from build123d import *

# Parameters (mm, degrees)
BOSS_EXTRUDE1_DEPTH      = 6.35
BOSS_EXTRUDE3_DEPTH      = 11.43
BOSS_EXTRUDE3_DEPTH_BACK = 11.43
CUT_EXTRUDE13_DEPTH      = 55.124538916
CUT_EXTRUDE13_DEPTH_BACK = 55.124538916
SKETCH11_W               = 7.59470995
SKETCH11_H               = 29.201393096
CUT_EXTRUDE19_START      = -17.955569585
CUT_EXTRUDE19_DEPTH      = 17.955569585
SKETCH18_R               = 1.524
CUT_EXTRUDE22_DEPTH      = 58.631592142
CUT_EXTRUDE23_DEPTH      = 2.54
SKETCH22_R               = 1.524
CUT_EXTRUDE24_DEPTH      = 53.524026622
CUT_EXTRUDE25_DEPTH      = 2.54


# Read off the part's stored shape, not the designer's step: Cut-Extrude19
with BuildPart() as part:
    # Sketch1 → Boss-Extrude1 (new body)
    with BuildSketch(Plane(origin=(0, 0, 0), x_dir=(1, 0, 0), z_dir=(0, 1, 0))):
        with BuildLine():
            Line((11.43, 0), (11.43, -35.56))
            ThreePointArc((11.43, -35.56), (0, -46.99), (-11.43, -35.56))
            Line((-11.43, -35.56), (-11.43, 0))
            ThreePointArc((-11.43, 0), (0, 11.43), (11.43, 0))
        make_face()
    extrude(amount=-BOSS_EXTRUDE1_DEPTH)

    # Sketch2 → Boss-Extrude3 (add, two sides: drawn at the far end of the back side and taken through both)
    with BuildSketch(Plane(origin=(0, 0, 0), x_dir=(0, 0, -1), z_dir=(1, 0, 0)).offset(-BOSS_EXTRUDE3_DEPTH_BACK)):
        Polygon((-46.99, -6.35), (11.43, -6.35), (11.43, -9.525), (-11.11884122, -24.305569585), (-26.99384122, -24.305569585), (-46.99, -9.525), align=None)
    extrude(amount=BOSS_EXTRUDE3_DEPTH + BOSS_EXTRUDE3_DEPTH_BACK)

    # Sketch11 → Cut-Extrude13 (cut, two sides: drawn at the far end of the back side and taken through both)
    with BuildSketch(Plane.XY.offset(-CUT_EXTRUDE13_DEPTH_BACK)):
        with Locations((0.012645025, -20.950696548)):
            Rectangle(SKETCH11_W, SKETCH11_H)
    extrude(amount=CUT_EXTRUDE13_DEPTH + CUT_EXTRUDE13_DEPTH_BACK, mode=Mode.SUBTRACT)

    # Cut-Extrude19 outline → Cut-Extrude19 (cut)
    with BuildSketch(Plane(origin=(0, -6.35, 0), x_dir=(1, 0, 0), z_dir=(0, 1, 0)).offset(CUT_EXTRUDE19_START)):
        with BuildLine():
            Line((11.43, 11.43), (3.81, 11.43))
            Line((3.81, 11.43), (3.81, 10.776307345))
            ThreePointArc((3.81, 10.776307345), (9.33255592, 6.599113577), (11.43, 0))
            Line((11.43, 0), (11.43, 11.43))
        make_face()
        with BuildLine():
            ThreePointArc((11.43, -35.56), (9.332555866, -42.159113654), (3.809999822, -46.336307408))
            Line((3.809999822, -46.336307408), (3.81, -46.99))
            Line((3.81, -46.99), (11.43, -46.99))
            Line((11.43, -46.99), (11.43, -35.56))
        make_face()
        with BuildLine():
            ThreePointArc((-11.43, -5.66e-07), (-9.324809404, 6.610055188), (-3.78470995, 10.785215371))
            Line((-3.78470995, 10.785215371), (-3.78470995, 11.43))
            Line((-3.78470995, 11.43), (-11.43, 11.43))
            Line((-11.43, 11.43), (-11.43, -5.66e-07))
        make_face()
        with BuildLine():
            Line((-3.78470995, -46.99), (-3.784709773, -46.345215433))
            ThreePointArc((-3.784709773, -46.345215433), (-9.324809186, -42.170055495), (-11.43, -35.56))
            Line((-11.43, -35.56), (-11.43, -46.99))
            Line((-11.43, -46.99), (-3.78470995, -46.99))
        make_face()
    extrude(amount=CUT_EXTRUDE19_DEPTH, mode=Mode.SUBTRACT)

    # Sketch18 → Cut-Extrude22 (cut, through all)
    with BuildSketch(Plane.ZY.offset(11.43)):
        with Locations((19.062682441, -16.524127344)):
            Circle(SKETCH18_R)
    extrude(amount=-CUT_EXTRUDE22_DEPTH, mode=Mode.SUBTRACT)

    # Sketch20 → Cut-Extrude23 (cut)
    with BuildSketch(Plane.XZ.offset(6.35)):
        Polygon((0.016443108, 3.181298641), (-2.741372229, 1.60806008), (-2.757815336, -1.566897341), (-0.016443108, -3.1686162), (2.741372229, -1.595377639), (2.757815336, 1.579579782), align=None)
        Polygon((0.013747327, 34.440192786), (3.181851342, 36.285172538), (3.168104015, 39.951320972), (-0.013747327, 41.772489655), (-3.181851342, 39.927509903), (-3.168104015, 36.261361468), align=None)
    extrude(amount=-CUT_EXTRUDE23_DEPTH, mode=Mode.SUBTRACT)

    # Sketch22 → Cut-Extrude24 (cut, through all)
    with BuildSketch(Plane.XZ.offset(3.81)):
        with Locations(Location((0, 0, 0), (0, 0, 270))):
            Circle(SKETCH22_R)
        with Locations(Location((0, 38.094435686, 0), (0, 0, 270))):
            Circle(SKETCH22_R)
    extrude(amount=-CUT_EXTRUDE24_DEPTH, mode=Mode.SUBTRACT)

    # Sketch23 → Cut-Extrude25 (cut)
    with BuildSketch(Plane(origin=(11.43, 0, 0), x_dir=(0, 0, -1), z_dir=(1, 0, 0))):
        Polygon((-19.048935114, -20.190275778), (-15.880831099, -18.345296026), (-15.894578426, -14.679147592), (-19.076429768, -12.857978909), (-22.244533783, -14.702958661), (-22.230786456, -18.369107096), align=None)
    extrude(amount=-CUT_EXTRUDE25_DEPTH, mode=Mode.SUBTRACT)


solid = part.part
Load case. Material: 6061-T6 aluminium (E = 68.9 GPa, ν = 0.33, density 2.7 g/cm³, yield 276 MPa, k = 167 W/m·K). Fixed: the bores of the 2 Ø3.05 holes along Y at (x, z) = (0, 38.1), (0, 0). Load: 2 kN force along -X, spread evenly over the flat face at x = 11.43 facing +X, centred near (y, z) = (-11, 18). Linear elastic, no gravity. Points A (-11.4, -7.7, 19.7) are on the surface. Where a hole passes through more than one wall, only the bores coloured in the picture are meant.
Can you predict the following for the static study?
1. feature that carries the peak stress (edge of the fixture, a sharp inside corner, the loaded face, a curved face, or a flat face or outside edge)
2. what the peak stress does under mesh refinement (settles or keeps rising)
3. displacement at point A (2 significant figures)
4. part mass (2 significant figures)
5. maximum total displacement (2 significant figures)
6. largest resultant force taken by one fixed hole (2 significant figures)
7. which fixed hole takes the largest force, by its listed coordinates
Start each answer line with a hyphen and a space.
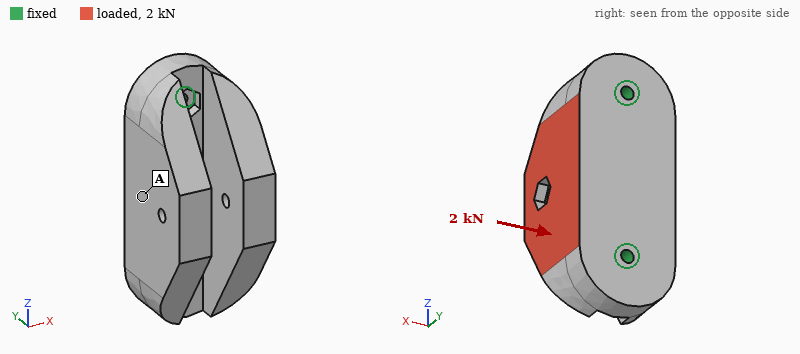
- edge of the fixture
- keeps rising
- 0.046 mm
- 49 g
- 0.13 mm
- 1.1 kN
- (0, 0)
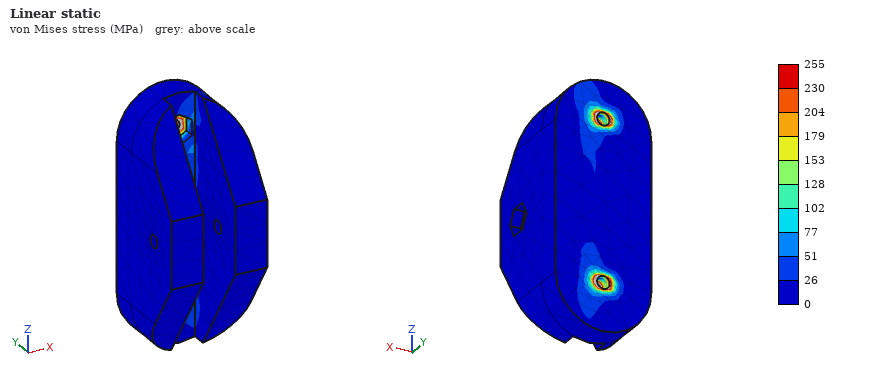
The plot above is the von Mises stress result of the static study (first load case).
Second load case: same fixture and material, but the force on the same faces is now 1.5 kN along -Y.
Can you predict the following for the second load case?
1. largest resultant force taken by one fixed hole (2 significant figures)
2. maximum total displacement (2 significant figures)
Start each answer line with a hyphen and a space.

- 840 N
- 0.11 mm
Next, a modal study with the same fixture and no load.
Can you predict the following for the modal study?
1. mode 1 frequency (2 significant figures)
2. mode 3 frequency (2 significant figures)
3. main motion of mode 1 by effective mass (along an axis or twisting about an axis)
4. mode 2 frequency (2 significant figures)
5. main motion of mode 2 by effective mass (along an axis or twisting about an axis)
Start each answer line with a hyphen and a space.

- 4000 Hz
- 14 kHz
- along X
- 9800 Hz
- along Y
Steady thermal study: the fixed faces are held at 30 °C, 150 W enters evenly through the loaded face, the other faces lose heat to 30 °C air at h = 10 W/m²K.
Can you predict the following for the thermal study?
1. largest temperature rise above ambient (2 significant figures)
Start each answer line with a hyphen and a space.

- 68 K
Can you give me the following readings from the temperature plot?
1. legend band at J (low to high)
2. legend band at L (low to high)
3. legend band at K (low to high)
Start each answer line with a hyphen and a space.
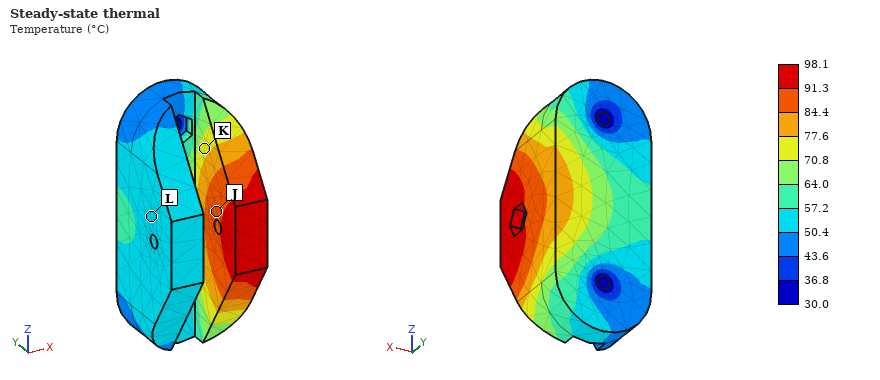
- 84.4 to 91.3 °C
- 50.4 to 57.2 °C
- 70.8 to 77.6 °C
